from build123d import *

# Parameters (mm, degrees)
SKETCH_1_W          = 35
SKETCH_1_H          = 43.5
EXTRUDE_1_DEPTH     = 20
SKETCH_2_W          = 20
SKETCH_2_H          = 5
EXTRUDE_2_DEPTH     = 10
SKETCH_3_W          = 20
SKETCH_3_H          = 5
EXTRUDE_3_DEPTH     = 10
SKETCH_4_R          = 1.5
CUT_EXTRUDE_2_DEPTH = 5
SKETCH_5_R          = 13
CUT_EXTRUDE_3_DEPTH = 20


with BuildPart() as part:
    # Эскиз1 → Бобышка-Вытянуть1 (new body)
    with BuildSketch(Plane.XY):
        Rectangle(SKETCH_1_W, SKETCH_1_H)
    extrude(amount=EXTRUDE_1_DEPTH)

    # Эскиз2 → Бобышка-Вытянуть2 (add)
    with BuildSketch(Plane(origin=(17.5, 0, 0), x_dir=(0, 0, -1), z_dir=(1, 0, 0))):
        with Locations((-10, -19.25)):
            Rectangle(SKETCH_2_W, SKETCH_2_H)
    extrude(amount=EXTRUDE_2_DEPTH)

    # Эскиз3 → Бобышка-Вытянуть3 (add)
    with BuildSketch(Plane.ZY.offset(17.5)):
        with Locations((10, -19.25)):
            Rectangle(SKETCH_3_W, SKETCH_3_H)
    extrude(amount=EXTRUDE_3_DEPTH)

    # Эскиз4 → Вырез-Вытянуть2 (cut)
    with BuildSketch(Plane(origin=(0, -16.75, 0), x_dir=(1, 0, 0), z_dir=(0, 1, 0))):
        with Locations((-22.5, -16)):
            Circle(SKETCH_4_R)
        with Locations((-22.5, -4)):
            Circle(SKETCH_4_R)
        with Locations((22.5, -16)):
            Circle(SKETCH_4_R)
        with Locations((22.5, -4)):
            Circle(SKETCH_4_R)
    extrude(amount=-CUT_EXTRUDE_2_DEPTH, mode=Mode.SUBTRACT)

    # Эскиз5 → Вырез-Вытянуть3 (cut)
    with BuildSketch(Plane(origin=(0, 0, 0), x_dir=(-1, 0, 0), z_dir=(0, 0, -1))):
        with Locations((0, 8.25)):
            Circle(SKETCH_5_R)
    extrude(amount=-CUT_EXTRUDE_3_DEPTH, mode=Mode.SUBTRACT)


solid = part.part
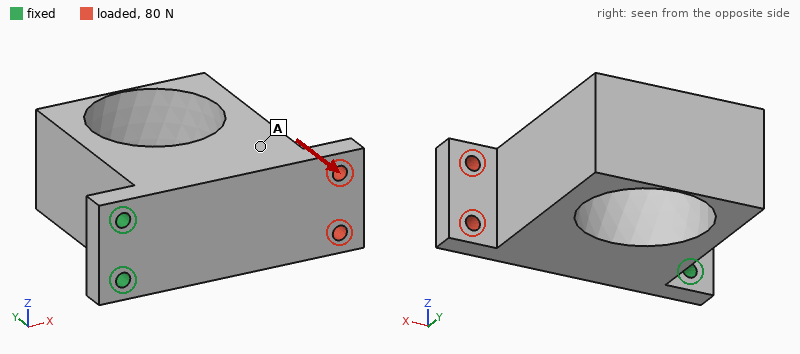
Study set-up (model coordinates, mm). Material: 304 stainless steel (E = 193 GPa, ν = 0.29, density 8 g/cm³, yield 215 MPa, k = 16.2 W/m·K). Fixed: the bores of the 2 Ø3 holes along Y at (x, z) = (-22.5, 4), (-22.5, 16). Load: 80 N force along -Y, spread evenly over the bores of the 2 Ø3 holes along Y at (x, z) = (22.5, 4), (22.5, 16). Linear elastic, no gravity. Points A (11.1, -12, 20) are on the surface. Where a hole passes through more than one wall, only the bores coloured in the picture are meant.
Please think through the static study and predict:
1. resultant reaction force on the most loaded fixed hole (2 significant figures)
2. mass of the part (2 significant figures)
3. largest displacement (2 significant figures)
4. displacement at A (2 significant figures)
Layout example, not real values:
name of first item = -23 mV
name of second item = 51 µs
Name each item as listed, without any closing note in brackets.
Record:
resultant reaction force on the most loaded fixed hole = 40 N
mass of the part = 170 g
largest displacement = 34 µm
displacement at A = 19 µm
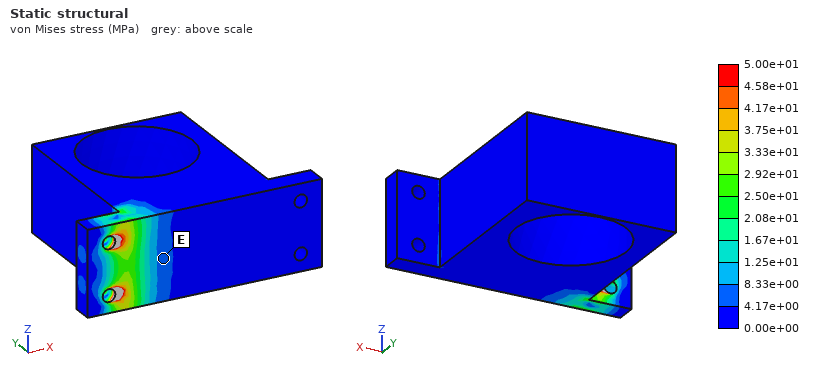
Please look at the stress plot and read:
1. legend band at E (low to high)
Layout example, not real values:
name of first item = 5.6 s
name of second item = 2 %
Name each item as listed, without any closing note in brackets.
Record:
legend band at E = 4.17e+00 to 8.33e+00 MPa
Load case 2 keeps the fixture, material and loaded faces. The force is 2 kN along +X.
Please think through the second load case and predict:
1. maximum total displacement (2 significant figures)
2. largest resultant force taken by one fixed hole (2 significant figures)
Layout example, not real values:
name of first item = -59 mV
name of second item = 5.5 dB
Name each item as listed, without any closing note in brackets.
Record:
maximum total displacement = 11 µm
largest resultant force taken by one fixed hole = 1.0 kN
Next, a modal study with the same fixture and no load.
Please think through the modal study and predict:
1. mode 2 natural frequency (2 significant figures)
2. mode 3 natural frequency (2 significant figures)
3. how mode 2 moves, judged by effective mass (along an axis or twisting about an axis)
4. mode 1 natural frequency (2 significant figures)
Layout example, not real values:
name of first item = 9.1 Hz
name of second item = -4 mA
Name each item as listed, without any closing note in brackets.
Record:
mode 2 natural frequency = 2600 Hz
mode 3 natural frequency = 4400 Hz
how mode 2 moves, judged by effective mass = along Z
mode 1 natural frequency = 940 Hz
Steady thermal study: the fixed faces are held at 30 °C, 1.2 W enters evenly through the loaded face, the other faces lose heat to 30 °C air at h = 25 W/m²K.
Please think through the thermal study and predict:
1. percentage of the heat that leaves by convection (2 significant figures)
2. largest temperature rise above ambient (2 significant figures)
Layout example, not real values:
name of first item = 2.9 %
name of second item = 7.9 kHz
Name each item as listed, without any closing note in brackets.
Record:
percentage of the heat that leaves by convection = 61 %
largest temperature rise above ambient = 13 K
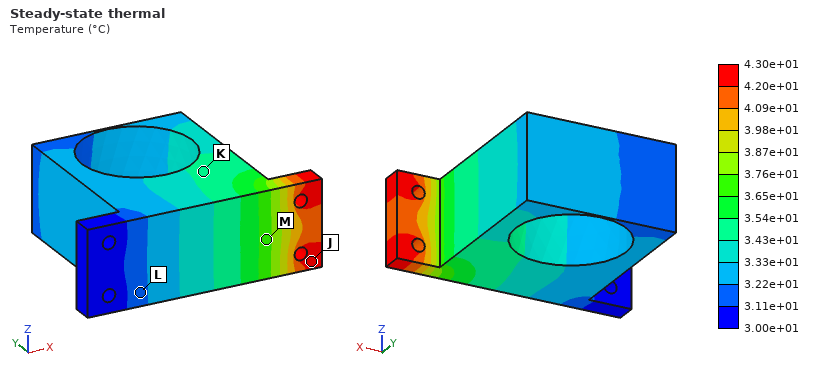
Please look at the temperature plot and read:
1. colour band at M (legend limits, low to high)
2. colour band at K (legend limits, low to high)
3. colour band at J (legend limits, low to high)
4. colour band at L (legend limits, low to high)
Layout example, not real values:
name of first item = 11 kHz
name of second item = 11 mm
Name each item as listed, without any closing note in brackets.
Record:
colour band at M = 3.65e+01 to 3.76e+01 °C
colour band at K = 3.43e+01 to 3.54e+01 °C
colour band at J = 4.20e+01 to 4.30e+01 °C
colour band at L = 3.11e+01 to 3.22e+01 °C
